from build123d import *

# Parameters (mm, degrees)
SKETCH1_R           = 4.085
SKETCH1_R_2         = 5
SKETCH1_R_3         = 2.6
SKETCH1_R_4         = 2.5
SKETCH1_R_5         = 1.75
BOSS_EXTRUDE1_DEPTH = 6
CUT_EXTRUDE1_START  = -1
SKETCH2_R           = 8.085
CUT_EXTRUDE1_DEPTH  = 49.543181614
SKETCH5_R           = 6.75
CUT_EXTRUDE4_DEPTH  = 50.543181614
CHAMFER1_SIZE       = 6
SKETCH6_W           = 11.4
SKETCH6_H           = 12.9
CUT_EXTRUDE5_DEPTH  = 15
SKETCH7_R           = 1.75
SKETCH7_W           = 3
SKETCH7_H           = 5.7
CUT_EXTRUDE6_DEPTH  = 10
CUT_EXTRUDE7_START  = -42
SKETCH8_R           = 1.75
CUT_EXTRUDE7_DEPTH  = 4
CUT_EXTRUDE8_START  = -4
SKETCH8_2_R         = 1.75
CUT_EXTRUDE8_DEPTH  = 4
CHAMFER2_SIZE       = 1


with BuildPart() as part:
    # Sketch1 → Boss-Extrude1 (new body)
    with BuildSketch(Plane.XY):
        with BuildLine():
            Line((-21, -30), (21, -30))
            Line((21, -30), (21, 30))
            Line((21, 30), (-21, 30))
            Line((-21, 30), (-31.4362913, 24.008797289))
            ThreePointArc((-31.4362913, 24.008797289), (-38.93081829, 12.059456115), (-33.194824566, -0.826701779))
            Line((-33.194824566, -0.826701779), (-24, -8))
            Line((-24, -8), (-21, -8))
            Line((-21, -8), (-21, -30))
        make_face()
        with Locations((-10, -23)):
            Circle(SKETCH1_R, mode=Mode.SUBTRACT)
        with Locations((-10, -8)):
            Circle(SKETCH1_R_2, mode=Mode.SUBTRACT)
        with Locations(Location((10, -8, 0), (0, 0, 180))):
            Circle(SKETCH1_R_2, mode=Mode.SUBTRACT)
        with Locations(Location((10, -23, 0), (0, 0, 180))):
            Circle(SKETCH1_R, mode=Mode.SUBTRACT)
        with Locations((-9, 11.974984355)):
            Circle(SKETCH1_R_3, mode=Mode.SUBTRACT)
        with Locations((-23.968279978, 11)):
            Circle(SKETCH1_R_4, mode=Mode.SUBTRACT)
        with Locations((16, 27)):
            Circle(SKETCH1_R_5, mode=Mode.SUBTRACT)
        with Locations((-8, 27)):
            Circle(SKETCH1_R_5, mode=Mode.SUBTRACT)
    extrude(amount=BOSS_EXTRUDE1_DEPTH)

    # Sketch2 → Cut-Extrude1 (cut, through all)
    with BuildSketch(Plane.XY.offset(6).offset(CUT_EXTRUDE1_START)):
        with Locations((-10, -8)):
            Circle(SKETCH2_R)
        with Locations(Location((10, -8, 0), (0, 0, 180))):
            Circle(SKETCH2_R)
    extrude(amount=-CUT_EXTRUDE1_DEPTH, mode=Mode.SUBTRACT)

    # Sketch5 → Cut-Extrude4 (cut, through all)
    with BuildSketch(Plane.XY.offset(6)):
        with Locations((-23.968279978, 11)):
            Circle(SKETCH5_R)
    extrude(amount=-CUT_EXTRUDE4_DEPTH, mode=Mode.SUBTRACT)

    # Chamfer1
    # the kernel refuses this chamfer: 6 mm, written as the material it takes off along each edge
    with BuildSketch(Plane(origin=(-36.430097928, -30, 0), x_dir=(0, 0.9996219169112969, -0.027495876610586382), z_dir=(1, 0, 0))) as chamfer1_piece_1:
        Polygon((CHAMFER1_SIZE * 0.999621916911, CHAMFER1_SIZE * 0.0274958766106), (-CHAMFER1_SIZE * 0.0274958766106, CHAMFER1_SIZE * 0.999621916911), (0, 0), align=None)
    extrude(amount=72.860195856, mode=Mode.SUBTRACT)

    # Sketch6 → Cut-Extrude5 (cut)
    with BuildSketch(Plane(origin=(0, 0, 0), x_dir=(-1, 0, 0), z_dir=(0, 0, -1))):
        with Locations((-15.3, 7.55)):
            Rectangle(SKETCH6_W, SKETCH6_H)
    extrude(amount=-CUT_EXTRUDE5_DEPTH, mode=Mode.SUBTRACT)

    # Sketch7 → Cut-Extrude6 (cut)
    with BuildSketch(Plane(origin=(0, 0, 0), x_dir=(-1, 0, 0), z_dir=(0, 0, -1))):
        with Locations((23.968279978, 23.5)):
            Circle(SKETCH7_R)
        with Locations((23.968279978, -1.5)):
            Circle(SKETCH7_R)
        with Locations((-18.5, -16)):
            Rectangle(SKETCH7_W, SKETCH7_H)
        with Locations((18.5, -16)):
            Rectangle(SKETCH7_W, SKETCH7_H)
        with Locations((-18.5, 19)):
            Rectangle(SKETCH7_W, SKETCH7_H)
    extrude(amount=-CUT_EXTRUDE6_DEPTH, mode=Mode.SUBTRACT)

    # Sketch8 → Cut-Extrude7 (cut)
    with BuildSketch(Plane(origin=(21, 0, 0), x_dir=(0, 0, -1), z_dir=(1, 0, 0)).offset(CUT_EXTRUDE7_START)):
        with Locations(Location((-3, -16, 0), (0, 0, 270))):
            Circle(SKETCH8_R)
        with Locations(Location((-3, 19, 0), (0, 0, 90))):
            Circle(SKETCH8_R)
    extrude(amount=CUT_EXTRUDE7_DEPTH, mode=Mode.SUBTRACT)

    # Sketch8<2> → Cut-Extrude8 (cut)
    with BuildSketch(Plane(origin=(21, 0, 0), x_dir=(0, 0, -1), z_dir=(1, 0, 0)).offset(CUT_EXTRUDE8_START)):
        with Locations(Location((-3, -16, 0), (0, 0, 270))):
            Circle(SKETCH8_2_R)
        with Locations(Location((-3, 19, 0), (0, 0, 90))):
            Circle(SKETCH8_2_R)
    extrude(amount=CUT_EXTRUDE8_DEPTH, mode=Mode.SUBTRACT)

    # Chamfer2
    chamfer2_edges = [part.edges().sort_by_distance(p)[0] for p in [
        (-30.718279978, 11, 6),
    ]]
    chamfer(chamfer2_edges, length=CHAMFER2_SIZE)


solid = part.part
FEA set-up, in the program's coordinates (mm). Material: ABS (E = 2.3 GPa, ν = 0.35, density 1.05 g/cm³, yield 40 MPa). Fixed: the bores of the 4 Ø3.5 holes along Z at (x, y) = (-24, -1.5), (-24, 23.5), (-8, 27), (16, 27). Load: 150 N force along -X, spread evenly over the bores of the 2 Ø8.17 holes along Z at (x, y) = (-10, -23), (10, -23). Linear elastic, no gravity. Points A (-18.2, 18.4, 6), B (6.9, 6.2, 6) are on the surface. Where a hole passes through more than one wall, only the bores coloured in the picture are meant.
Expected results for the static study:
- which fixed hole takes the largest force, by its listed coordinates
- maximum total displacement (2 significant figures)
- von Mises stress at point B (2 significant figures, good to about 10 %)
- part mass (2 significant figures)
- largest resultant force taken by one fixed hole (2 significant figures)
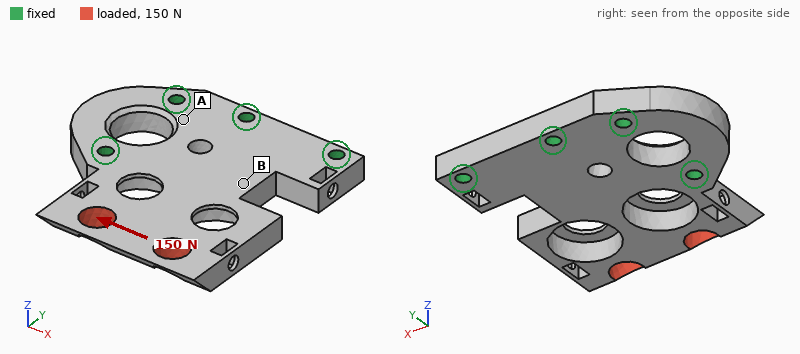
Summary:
(-24, -1.5)
0.28 mm
3.1 MPa
13 g
170 N
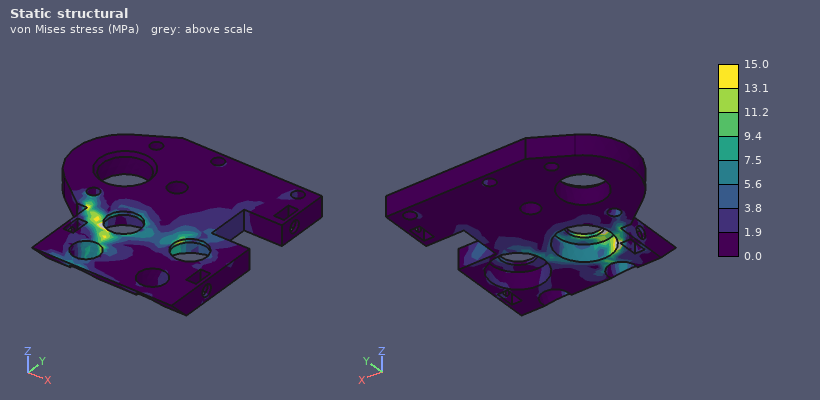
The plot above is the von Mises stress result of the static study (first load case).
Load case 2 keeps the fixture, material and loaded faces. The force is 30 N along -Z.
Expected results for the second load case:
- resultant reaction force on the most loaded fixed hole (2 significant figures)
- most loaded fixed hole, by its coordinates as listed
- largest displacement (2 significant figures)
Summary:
34 N
(-24, -1.5)
0.99 mm
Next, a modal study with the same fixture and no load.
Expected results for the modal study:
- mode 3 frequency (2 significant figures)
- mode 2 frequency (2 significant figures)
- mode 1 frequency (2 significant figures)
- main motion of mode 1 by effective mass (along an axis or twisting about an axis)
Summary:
2600 Hz
1800 Hz
690 Hz
along Z
